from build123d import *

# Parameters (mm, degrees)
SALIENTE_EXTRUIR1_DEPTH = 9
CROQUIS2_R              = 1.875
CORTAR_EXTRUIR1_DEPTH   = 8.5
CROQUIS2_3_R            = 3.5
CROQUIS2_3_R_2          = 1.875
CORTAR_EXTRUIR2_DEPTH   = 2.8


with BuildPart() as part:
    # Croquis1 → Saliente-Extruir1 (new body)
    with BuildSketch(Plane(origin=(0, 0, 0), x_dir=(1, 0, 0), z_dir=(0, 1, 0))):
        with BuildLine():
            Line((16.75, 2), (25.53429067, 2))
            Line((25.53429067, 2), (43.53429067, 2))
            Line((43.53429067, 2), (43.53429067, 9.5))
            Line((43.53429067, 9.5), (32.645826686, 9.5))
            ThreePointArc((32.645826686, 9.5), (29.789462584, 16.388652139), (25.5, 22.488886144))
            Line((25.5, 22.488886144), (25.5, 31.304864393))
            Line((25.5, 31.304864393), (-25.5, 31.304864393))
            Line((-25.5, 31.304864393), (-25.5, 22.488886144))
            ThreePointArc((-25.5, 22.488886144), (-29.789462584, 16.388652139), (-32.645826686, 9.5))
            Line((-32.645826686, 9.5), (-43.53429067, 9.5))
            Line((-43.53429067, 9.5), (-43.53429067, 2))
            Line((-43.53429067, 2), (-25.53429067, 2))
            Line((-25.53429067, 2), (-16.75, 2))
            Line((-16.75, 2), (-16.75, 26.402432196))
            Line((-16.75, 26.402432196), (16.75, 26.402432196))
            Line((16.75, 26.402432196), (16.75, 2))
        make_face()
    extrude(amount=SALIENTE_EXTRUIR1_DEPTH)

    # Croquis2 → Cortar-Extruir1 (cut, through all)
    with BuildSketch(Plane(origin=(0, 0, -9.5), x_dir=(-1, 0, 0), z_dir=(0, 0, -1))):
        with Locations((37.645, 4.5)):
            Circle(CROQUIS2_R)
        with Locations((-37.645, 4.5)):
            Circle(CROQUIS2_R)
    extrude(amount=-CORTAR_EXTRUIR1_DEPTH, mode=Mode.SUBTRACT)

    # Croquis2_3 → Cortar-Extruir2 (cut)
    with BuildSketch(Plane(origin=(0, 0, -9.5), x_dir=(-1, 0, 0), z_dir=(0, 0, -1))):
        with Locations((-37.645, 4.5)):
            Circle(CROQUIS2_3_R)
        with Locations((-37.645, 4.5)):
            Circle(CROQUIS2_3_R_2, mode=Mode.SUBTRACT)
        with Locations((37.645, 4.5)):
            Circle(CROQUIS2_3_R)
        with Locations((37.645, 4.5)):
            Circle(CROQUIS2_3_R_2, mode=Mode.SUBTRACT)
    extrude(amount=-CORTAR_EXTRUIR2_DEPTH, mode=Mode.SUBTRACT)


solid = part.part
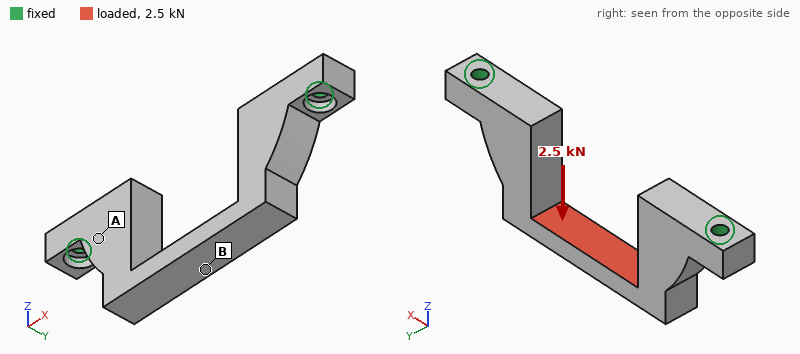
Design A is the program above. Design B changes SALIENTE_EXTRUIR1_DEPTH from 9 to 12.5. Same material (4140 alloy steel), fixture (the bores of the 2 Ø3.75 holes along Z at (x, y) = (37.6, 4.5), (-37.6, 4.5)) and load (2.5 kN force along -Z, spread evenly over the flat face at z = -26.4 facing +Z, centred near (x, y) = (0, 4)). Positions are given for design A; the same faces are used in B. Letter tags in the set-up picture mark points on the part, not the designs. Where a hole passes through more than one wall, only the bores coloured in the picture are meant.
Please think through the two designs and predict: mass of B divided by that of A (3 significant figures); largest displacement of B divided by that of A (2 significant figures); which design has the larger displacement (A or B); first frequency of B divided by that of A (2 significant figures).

1.40
0.81
A
1.0
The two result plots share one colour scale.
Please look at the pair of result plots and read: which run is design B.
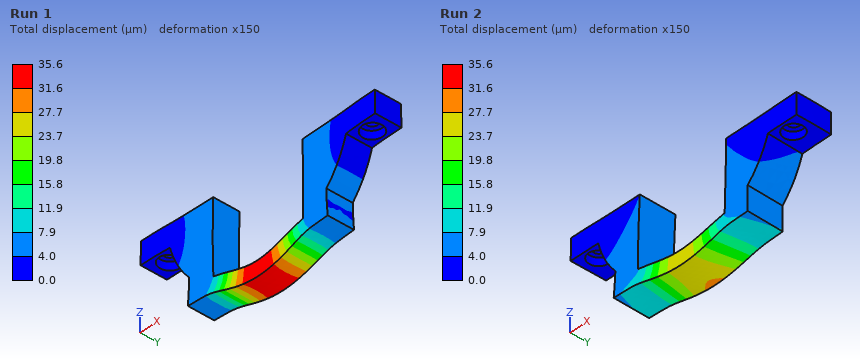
Run 2
